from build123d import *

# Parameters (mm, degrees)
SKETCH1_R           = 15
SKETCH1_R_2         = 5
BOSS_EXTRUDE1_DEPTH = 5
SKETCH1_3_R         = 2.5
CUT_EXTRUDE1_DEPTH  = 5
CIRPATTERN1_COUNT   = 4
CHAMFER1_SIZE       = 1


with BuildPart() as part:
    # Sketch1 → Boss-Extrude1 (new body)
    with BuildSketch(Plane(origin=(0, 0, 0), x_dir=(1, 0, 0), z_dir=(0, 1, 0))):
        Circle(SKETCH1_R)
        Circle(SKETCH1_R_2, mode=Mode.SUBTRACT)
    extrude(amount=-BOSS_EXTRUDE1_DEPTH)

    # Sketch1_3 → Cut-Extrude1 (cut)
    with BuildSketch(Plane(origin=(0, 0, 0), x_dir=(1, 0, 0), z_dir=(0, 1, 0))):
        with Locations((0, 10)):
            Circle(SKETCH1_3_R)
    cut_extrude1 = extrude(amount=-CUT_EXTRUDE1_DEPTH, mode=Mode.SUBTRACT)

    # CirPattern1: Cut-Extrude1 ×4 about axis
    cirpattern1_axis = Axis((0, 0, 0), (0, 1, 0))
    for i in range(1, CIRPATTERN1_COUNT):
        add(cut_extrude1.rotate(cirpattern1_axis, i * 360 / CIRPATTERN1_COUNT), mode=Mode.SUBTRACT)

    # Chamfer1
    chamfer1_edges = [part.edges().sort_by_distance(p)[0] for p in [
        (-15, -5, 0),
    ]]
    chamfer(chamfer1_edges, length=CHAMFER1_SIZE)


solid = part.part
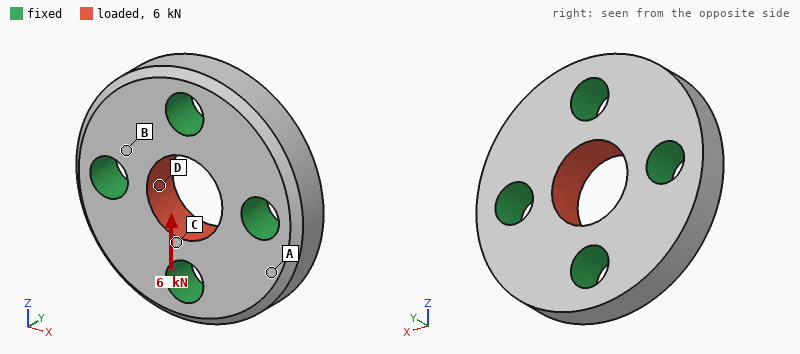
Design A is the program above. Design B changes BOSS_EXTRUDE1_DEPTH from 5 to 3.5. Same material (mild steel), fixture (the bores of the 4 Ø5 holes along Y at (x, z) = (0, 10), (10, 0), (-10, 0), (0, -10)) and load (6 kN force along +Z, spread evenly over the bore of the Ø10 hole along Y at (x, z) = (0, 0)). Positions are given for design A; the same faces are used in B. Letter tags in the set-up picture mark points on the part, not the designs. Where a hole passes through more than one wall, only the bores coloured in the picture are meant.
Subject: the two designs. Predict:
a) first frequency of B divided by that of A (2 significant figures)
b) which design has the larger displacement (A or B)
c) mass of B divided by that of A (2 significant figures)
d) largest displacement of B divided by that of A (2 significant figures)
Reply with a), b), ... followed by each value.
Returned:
a) 0.84
b) B
c) 0.69
d) 1.4
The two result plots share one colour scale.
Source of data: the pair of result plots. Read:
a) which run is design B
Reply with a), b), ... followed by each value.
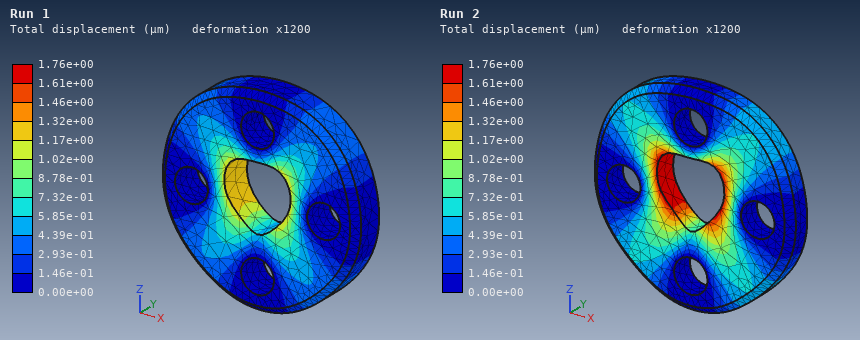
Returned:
a) Run 2
